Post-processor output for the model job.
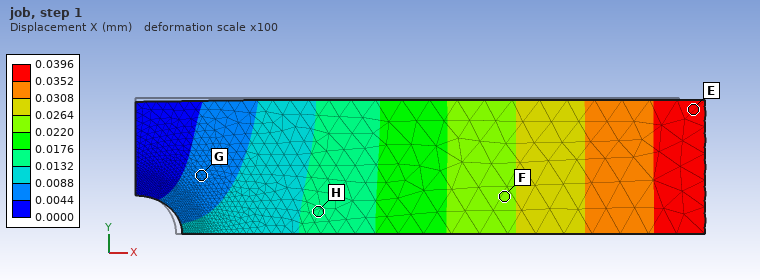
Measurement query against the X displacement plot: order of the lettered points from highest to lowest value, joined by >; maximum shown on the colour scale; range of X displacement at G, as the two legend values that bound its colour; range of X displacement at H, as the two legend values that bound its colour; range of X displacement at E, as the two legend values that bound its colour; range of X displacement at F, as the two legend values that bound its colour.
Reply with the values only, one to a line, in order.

E > F > H > G
0.0396 mm
0.0044 to 0.0088 mm
0.0132 to 0.0176 mm
0.0352 to 0.0396 mm
0.0220 to 0.0264 mm
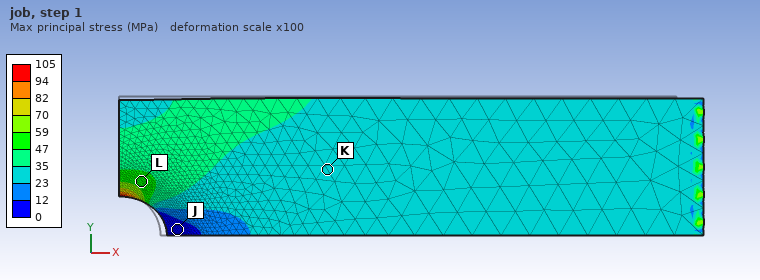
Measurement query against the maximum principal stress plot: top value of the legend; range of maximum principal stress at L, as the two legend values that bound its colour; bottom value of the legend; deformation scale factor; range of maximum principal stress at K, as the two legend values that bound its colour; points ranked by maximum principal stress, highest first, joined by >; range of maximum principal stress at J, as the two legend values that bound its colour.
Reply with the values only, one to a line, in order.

105 MPa
47 to 59 MPa
0 MPa
100
23 to 35 MPa
L > K > J
0 to 12 MPa
